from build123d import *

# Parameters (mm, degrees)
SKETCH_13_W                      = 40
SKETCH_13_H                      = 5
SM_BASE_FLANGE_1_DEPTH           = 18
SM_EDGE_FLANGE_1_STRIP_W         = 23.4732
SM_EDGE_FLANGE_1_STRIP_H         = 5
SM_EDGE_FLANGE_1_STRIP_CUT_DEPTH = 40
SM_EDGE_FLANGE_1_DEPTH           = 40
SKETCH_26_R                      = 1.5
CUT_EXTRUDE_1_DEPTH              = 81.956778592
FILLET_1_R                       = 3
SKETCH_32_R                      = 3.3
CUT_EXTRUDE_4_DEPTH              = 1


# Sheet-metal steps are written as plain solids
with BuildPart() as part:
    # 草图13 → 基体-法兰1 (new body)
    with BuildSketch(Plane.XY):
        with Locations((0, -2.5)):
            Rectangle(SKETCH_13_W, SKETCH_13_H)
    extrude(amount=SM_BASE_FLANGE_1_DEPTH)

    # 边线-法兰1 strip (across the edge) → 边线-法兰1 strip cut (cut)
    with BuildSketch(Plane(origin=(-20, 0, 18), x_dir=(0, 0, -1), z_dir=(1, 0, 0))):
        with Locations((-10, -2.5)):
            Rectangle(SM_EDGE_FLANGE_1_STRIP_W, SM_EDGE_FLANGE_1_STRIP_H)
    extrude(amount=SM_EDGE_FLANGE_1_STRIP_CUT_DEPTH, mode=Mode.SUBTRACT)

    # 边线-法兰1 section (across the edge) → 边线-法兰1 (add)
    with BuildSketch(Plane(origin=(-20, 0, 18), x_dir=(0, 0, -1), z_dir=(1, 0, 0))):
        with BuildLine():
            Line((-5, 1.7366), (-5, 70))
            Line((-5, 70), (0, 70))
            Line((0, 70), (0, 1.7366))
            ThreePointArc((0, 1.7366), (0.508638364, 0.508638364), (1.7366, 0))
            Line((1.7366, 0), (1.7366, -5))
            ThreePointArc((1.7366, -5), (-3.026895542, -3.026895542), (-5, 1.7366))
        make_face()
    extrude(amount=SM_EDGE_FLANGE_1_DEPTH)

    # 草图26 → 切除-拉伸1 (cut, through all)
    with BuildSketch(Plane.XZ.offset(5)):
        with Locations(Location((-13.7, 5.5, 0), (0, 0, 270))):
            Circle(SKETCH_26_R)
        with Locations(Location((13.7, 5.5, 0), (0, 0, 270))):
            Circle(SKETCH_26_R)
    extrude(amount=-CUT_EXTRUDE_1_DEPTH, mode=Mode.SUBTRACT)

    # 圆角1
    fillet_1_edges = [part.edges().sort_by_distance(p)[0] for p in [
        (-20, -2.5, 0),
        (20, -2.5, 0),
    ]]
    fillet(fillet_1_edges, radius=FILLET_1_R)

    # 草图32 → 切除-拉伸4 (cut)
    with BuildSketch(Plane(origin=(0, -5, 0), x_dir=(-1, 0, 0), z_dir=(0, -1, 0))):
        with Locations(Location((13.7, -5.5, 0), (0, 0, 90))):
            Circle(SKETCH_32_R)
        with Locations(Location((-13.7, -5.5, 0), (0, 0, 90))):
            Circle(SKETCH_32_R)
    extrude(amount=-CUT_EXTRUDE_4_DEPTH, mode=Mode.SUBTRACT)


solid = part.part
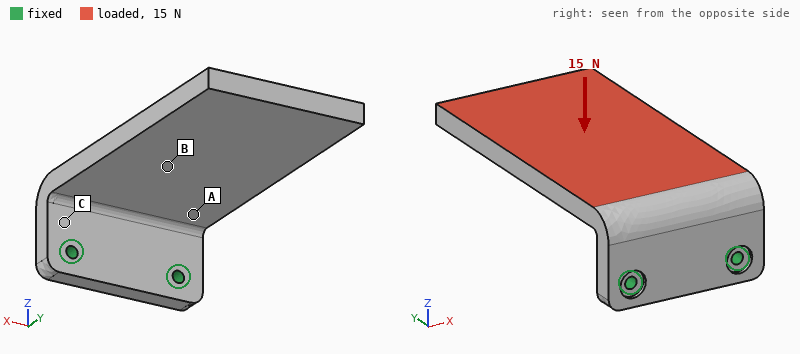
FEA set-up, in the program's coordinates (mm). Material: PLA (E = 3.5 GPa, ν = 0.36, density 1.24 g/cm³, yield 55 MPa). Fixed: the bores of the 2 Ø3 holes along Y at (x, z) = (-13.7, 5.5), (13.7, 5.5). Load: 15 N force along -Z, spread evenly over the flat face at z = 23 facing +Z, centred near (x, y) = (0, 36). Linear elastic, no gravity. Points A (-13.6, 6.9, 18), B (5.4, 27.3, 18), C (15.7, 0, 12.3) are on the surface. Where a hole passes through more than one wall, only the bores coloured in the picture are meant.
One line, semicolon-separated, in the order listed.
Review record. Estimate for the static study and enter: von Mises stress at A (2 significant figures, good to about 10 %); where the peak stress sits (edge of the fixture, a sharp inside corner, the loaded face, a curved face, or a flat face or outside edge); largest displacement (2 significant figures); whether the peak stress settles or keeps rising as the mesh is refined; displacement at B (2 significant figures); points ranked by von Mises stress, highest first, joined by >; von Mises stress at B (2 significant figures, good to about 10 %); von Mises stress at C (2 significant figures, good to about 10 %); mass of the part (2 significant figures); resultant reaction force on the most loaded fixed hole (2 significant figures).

2.4 MPa; edge of the fixture; 0.98 mm; keeps rising; 0.33 mm; C > A > B; 1.2 MPa; 3.6 MPa; 22 g; 8.7 N
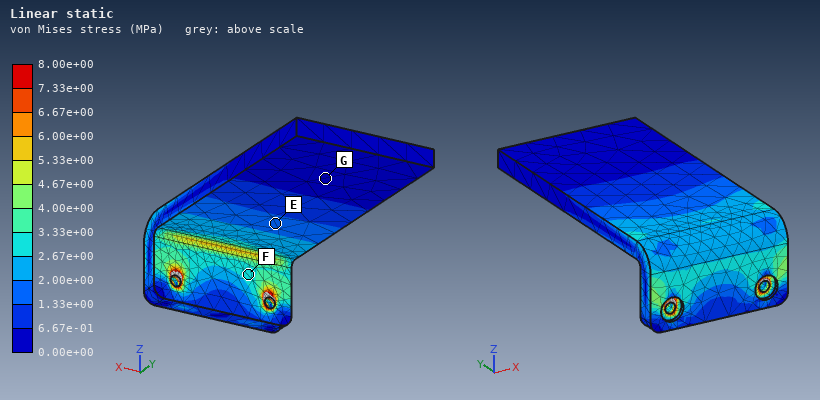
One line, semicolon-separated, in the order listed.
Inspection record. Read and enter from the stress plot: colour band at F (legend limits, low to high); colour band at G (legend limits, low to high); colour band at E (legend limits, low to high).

2.67e+00 to 3.33e+00 MPa; 0.00e+00 to 6.67e-01 MPa; 1.33e+00 to 2.00e+00 MPa
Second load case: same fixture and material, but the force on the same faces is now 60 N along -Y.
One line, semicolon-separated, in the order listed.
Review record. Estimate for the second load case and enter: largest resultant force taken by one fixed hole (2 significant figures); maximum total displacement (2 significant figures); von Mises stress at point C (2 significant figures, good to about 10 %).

30 N; 0.85 mm; 4.1 MPa
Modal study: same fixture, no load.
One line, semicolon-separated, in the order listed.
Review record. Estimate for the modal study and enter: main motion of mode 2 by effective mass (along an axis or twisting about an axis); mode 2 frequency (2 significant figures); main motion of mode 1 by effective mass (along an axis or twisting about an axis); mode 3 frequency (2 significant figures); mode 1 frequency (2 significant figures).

along X; 490 Hz; along Z; 950 Hz; 190 Hz
